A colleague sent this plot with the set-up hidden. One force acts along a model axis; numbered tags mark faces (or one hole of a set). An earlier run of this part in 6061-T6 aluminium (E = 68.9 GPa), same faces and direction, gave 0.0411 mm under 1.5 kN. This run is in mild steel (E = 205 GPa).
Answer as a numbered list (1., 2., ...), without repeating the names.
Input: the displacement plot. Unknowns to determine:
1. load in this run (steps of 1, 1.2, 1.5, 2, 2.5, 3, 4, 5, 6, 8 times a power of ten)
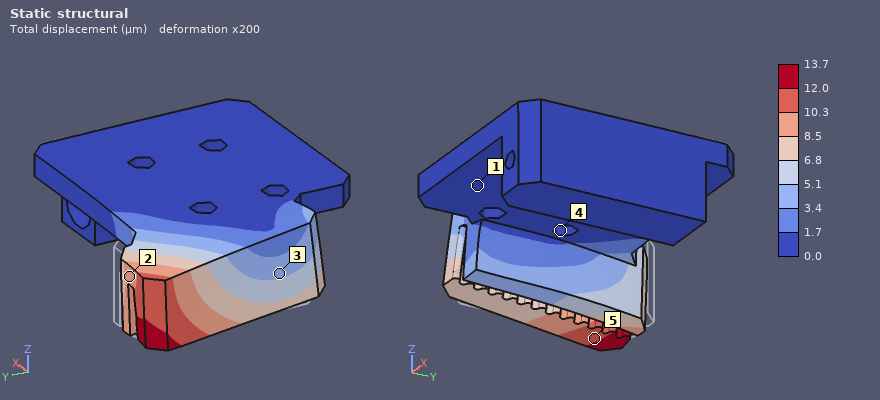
1. 1.5 kN
